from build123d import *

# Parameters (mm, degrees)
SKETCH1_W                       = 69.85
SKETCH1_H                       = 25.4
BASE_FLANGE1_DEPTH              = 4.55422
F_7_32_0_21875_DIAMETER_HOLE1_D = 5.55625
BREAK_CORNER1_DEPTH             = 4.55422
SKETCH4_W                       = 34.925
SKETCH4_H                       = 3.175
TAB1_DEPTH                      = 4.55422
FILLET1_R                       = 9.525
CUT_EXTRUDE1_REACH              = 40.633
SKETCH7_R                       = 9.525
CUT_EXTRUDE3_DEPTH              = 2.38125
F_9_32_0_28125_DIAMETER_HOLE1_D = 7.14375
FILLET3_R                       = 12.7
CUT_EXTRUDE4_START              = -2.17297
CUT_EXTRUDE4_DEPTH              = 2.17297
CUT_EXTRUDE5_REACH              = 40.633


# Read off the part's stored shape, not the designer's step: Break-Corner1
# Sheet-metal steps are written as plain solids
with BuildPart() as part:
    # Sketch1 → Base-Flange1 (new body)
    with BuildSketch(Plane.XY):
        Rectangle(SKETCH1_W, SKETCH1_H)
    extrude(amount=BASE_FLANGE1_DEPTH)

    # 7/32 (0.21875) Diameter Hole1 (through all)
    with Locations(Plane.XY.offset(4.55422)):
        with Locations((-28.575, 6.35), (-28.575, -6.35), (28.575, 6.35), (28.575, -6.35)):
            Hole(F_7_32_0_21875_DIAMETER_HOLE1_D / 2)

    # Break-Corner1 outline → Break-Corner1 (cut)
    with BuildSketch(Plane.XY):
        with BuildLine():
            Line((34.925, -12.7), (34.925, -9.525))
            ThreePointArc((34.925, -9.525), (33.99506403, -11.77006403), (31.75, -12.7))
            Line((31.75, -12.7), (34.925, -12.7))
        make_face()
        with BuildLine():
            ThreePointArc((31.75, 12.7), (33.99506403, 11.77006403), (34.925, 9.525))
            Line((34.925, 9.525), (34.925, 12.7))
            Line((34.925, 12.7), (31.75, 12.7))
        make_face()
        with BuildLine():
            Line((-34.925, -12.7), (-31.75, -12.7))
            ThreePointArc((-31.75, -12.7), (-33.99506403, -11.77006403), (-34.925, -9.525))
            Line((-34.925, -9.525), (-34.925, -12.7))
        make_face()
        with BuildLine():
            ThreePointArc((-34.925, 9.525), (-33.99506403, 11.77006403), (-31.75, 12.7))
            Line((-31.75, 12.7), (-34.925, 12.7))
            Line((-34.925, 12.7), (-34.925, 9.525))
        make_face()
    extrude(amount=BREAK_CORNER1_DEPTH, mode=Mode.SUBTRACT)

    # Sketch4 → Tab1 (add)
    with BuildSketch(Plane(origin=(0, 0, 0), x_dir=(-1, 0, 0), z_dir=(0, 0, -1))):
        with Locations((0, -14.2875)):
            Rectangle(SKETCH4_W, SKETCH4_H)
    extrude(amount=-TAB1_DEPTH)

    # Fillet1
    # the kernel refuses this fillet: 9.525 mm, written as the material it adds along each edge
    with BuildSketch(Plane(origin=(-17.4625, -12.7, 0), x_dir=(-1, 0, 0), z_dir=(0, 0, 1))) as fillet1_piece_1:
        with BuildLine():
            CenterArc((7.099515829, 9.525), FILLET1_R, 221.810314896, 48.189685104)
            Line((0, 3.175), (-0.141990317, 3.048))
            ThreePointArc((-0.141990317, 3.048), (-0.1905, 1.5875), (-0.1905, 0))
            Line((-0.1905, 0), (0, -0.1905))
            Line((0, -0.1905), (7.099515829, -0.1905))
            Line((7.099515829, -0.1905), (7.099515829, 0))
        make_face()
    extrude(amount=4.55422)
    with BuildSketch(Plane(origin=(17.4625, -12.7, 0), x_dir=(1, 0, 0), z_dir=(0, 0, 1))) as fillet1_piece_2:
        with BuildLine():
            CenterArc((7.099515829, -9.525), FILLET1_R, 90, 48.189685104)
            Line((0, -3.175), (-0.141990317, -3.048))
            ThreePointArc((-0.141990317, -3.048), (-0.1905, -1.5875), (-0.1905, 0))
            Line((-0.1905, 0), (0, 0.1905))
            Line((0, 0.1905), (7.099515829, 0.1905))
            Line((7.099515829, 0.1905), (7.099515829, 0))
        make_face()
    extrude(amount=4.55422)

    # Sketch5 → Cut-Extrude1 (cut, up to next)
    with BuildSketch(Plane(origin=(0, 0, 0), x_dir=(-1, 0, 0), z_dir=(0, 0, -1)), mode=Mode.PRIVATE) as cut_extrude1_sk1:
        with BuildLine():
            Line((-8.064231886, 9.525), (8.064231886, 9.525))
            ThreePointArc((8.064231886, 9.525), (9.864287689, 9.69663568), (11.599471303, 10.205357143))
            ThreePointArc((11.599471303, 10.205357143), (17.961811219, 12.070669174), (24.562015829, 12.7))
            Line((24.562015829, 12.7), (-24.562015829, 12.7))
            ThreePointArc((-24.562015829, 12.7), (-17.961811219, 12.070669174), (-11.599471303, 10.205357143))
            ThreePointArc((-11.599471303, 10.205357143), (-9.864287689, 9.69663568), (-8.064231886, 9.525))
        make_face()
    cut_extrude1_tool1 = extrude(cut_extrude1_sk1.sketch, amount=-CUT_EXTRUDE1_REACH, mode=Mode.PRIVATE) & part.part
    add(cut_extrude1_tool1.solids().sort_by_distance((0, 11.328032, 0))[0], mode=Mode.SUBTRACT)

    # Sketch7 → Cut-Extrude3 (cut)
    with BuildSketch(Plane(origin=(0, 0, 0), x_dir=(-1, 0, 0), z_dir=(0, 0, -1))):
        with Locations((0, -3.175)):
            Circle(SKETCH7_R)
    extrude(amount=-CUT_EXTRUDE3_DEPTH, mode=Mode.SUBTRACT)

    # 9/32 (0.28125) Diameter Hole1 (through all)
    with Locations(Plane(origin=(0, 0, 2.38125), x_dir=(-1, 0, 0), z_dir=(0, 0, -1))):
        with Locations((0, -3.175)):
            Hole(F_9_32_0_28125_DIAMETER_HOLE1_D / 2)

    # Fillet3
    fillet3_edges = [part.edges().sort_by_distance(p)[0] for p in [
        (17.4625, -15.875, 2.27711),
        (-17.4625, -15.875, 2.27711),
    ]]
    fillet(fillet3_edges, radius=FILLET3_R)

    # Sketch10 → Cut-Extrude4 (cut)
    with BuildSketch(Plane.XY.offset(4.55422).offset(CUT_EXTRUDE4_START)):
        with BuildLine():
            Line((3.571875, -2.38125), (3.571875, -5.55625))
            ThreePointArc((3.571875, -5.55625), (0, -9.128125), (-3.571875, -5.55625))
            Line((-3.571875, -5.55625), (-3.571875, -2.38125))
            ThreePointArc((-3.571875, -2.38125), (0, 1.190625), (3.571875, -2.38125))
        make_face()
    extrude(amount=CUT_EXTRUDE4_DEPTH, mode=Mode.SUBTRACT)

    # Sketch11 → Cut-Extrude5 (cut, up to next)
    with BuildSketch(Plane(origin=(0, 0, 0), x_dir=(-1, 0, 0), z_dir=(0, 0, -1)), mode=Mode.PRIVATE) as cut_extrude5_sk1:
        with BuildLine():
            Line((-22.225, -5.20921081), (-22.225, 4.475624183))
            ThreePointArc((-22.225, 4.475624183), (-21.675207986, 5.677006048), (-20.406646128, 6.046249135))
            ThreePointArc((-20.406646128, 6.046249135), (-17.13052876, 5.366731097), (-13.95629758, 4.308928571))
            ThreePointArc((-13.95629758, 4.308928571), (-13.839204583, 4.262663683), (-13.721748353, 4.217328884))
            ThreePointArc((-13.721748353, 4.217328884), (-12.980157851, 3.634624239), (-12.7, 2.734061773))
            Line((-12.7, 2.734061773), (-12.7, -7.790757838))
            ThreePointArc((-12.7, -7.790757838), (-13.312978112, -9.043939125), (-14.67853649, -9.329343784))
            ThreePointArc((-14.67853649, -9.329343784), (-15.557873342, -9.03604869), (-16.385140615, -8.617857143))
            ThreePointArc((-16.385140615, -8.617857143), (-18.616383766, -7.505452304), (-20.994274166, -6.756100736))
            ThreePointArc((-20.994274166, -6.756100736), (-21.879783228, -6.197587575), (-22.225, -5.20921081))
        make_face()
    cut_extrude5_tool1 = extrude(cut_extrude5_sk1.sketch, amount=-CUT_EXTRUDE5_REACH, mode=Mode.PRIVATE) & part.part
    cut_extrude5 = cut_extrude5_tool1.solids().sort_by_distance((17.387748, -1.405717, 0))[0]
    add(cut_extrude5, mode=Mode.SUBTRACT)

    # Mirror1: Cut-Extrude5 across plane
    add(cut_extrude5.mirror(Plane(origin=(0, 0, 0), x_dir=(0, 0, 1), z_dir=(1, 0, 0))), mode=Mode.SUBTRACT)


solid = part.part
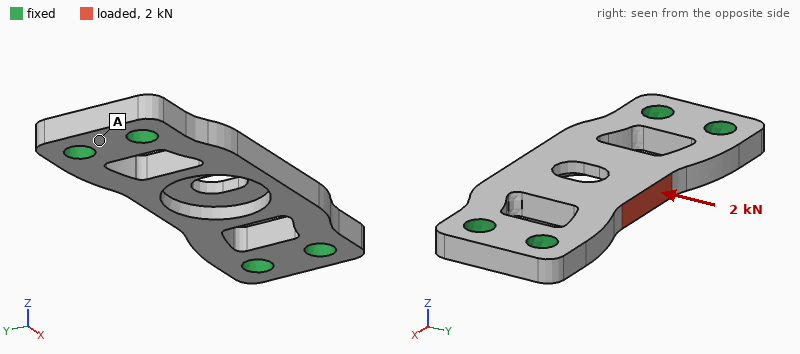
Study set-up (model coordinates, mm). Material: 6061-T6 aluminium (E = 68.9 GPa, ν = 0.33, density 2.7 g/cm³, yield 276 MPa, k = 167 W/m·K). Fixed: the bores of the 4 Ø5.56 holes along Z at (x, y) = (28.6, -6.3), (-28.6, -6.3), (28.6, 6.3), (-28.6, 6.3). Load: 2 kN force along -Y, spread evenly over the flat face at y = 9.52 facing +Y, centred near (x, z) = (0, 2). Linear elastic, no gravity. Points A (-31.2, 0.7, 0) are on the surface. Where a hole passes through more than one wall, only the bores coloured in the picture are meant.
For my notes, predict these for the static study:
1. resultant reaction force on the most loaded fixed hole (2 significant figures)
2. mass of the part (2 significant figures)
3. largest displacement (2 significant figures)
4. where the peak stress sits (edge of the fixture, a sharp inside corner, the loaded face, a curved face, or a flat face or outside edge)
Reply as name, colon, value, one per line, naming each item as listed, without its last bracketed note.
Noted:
resultant reaction force on the most loaded fixed hole: 770 N
mass of the part: 16 g
largest displacement: 60 µm
where the peak stress sits: a curved face
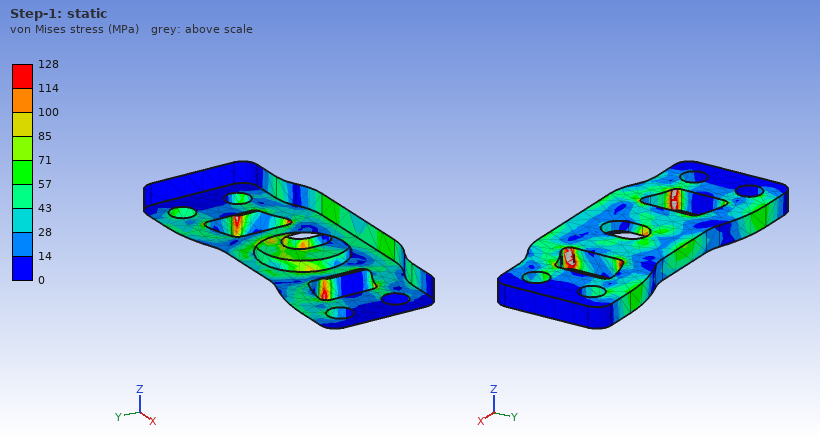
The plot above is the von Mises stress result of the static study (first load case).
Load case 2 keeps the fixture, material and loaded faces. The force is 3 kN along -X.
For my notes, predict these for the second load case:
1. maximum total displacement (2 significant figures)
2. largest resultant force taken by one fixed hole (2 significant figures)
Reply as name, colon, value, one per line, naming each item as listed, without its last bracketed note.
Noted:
maximum total displacement: 25 µm
largest resultant force taken by one fixed hole: 1.4 kN
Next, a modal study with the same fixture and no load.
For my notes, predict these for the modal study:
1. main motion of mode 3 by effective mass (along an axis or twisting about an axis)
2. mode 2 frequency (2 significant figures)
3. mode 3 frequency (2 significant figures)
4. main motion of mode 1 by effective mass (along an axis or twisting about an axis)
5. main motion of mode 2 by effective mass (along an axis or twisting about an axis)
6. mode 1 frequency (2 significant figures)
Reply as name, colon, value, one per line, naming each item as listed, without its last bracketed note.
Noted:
main motion of mode 3 by effective mass: along Y
mode 2 frequency: 10 kHz
mode 3 frequency: 15 kHz
main motion of mode 1 by effective mass: along Z
main motion of mode 2 by effective mass: twisting about X
mode 1 frequency: 6900 Hz
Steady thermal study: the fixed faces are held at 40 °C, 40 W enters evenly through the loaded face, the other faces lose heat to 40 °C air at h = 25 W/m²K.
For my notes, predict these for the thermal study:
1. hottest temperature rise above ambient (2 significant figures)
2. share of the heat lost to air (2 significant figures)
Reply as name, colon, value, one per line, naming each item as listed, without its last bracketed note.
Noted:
hottest temperature rise above ambient: 68 K
share of the heat lost to air: 4.5 %
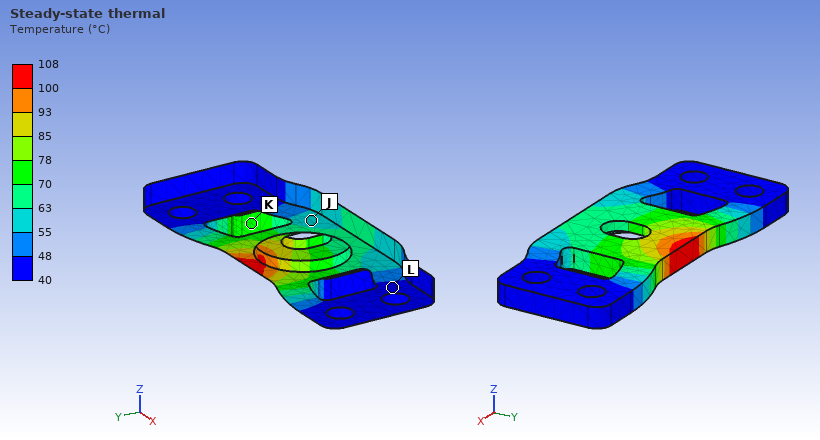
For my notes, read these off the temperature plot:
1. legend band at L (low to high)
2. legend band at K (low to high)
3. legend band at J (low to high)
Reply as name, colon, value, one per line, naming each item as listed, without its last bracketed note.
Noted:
legend band at L: 40 to 48 °C
legend band at K: 70 to 78 °C
legend band at J: 55 to 63 °C
